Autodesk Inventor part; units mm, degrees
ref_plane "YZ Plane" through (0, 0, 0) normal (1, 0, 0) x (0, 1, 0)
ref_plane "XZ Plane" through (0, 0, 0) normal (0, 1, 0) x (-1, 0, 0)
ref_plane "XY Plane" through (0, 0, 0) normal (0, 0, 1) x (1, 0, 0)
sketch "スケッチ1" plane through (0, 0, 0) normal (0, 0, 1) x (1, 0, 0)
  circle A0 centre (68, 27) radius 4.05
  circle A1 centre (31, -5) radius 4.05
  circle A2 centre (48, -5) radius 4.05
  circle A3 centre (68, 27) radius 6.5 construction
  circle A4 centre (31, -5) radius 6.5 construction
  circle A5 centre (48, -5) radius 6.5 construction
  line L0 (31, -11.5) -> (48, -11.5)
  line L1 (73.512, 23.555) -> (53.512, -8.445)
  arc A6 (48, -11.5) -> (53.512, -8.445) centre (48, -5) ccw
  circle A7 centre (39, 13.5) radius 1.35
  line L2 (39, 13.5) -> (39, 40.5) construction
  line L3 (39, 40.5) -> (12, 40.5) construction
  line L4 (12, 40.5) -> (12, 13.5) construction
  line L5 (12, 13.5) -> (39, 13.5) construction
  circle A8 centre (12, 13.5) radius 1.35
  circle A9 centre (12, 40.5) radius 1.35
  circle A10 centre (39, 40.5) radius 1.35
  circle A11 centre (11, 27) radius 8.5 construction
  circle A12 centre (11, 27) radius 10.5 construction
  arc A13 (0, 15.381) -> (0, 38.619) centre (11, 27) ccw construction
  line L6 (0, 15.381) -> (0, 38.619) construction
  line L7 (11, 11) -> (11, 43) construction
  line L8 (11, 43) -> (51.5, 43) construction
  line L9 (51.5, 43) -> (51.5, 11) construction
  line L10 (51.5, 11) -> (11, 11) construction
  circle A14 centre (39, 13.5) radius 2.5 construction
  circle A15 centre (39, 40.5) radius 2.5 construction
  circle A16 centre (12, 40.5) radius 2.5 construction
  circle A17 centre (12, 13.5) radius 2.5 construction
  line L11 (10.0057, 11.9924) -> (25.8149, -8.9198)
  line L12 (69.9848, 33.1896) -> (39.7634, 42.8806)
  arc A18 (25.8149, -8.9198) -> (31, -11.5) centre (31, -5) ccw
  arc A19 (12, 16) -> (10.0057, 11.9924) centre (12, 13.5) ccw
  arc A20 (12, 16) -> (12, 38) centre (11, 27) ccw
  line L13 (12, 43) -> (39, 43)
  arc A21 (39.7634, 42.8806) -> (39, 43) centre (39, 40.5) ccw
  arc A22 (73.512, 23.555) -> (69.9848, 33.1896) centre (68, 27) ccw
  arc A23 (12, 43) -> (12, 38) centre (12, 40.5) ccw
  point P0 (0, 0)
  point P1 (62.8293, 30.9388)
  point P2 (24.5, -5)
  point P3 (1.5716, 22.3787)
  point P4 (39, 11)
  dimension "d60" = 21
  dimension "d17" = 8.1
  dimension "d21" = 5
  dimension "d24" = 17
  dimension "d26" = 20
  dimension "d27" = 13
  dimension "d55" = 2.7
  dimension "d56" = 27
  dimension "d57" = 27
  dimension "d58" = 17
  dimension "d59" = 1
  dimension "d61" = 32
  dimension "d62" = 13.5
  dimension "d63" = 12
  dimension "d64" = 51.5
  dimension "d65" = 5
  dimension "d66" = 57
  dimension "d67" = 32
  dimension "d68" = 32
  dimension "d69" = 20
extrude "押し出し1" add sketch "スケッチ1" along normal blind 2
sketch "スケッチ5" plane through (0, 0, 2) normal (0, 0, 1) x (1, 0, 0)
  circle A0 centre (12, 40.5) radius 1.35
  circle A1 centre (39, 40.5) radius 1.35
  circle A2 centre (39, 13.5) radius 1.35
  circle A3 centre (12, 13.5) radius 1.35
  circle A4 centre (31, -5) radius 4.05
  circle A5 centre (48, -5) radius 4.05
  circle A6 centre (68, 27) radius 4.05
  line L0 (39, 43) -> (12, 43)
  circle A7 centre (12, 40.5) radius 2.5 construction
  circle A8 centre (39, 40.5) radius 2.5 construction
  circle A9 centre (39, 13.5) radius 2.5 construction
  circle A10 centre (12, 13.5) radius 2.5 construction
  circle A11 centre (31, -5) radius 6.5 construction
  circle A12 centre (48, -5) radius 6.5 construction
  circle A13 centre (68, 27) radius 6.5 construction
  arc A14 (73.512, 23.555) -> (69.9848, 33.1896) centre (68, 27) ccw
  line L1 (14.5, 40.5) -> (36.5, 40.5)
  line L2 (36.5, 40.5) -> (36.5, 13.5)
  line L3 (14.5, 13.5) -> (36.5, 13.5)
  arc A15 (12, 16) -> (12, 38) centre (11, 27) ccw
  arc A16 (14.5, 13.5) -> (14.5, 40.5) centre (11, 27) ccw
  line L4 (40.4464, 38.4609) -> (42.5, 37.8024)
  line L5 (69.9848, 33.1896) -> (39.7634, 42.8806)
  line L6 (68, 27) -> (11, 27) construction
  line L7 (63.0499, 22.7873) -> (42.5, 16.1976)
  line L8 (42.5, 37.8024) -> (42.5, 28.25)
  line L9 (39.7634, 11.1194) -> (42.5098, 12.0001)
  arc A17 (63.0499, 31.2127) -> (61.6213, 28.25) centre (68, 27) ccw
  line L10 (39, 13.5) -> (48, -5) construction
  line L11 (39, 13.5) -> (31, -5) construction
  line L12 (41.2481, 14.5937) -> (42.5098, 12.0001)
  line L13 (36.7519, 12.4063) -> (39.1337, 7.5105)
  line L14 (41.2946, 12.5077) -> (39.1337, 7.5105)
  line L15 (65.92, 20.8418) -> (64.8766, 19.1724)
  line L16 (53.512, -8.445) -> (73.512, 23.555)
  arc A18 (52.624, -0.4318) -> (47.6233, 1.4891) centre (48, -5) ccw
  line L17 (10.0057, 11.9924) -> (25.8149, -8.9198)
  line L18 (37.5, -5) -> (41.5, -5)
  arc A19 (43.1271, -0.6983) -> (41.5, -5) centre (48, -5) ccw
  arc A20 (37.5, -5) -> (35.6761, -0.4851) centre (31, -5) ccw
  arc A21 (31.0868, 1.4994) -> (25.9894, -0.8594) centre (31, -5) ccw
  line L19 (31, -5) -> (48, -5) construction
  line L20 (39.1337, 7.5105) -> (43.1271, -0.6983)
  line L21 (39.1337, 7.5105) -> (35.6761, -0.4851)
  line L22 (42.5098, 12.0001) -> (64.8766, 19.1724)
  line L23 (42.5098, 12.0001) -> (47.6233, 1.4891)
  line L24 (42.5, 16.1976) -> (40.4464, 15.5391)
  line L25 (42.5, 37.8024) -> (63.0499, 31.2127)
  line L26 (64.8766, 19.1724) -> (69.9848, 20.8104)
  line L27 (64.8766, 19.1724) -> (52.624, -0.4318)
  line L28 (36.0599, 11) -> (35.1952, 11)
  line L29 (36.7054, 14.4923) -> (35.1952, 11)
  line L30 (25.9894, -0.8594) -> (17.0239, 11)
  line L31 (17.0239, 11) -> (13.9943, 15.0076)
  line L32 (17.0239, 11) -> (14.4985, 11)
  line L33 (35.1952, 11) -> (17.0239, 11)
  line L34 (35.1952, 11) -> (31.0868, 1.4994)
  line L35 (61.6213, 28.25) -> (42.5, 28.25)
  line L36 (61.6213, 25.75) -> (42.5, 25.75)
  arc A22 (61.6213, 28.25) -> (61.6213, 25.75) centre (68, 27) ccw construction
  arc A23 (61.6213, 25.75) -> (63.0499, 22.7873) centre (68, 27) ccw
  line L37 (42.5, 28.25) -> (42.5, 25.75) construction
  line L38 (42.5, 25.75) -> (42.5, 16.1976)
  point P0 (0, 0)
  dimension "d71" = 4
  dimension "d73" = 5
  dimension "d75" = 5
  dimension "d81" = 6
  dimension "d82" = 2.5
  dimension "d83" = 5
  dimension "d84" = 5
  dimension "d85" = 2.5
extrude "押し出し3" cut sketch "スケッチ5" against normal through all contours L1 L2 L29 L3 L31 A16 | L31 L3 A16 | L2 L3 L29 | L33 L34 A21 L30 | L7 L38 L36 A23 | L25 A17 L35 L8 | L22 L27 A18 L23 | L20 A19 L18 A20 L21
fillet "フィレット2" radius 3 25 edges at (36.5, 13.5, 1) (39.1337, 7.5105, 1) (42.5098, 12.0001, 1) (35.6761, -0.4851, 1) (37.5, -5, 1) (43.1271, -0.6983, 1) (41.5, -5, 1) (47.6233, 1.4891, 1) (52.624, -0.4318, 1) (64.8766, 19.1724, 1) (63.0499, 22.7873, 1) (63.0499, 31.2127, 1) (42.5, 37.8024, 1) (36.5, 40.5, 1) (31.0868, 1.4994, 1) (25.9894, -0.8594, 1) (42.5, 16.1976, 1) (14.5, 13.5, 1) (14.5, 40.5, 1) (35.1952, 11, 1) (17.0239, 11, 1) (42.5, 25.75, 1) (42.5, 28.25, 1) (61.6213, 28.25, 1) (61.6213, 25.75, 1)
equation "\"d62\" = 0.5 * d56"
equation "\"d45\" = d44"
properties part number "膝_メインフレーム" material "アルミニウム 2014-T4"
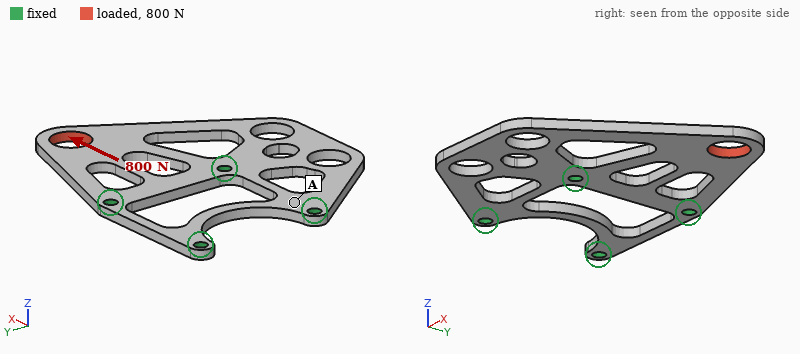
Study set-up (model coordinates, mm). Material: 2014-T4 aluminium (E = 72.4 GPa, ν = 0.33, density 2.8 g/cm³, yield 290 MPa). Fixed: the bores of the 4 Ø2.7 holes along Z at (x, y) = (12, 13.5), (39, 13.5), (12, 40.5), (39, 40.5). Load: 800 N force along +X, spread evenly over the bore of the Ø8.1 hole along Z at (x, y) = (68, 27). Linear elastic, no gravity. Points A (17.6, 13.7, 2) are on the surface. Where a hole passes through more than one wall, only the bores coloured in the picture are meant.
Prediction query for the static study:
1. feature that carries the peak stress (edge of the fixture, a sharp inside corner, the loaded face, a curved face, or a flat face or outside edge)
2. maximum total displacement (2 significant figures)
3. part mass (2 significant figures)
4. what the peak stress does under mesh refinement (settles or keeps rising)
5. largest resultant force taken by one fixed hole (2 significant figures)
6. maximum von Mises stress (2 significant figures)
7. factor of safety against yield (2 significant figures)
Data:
the loaded face
22 µm
8.0 g
settles
430 N
85 MPa
3.4
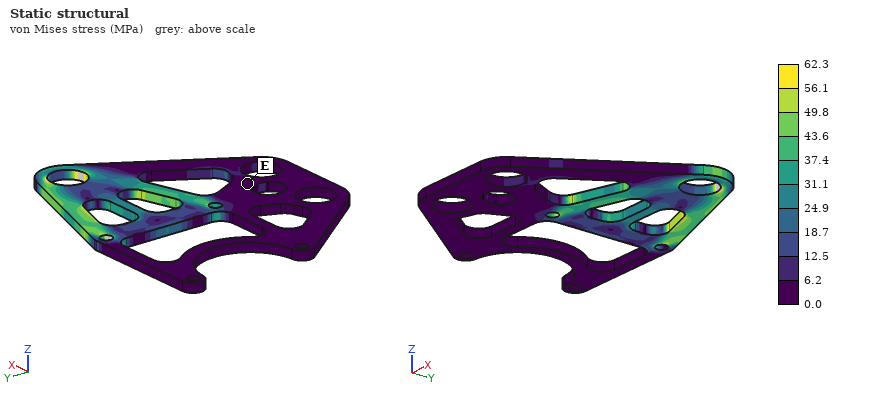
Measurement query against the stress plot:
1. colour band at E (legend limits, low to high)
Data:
0.0 to 6.2 MPa
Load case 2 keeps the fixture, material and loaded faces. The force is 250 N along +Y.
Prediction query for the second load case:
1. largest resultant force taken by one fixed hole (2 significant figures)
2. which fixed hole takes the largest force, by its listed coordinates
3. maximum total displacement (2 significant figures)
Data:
250 N
(39, 13.5)
26 µm
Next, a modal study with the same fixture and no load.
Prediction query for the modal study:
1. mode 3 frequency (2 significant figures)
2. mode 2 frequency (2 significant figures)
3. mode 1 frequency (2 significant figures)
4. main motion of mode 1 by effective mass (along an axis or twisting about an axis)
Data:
3900 Hz
2300 Hz
1400 Hz
along Z
